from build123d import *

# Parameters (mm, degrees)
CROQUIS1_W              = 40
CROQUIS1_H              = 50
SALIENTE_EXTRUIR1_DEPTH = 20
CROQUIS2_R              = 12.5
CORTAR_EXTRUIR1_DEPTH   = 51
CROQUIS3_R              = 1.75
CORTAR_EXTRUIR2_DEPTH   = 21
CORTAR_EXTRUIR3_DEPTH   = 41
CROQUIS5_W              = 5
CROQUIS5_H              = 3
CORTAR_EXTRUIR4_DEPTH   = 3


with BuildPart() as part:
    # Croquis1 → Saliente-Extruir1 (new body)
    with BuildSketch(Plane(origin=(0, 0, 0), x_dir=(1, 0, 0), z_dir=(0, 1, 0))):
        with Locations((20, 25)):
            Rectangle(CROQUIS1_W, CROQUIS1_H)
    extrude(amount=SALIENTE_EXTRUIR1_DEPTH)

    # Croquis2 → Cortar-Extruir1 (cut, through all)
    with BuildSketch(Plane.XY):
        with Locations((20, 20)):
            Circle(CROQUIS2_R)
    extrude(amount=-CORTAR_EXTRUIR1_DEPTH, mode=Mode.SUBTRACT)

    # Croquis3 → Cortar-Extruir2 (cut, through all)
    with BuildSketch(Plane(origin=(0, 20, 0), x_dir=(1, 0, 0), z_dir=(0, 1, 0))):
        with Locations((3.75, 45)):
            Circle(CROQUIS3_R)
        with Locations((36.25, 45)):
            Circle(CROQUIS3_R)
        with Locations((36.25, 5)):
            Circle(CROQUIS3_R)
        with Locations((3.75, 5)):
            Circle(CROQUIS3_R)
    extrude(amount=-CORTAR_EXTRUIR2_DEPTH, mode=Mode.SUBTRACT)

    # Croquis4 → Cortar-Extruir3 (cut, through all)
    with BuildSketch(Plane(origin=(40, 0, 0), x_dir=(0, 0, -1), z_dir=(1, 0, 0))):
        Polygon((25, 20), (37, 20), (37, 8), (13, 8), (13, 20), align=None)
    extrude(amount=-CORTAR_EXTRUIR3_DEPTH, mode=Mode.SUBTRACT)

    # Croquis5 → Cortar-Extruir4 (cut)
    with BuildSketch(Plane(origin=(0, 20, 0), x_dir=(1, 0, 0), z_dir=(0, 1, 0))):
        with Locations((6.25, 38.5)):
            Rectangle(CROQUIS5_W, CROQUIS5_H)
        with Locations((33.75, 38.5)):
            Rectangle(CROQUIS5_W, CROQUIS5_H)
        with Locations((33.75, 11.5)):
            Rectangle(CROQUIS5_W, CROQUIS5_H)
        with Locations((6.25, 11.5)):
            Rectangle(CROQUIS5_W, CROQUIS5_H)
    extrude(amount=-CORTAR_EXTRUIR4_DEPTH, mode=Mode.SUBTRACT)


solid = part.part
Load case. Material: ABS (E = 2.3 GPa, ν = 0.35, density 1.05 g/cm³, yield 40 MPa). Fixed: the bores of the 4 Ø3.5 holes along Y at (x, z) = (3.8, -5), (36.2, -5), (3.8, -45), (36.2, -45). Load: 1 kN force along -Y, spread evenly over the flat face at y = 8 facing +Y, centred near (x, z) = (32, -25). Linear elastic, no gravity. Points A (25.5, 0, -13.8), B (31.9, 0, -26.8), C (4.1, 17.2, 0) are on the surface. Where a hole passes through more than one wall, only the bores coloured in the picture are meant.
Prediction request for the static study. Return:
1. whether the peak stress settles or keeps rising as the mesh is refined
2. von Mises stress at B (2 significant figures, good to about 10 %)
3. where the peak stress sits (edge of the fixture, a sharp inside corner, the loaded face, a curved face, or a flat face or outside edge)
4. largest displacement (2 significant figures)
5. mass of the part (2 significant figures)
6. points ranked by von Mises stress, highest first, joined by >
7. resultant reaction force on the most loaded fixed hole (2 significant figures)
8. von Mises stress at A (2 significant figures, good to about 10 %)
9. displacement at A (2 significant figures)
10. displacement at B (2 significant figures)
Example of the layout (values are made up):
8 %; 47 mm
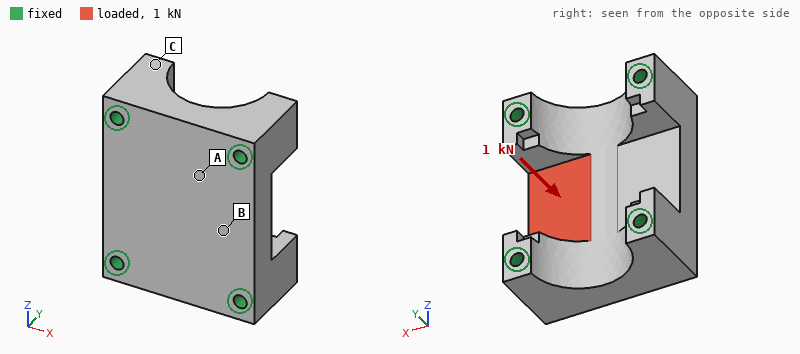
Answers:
keeps rising; 8.3 MPa; edge of the fixture; 0.14 mm; 22 g; B > A > C; 460 N; 3.1 MPa; 0.050 mm; 0.10 mm
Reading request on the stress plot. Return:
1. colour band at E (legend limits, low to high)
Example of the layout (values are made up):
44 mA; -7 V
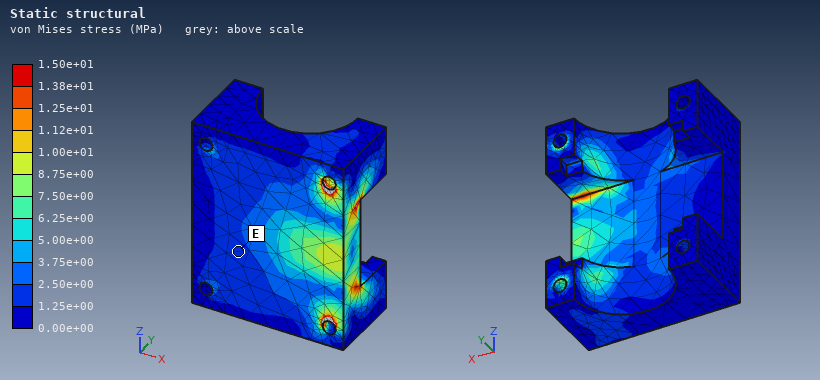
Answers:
1.25e+00 to 2.50e+00 MPa
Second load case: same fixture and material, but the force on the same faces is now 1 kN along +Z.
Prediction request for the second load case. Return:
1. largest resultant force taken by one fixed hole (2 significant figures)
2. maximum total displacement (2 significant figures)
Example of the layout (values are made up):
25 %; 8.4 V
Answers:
400 N; 36 µm
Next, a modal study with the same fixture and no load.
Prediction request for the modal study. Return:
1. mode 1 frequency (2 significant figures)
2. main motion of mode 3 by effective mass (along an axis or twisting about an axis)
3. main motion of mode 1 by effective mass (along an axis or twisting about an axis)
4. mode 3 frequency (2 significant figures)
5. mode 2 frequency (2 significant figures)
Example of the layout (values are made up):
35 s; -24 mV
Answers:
7100 Hz; along X; along Y; 10 kHz; 9200 Hz
